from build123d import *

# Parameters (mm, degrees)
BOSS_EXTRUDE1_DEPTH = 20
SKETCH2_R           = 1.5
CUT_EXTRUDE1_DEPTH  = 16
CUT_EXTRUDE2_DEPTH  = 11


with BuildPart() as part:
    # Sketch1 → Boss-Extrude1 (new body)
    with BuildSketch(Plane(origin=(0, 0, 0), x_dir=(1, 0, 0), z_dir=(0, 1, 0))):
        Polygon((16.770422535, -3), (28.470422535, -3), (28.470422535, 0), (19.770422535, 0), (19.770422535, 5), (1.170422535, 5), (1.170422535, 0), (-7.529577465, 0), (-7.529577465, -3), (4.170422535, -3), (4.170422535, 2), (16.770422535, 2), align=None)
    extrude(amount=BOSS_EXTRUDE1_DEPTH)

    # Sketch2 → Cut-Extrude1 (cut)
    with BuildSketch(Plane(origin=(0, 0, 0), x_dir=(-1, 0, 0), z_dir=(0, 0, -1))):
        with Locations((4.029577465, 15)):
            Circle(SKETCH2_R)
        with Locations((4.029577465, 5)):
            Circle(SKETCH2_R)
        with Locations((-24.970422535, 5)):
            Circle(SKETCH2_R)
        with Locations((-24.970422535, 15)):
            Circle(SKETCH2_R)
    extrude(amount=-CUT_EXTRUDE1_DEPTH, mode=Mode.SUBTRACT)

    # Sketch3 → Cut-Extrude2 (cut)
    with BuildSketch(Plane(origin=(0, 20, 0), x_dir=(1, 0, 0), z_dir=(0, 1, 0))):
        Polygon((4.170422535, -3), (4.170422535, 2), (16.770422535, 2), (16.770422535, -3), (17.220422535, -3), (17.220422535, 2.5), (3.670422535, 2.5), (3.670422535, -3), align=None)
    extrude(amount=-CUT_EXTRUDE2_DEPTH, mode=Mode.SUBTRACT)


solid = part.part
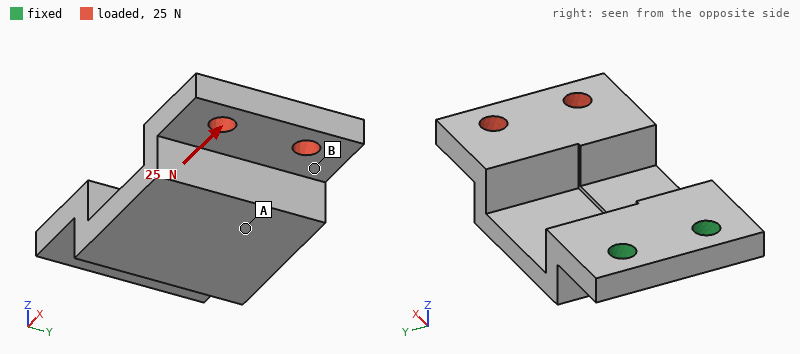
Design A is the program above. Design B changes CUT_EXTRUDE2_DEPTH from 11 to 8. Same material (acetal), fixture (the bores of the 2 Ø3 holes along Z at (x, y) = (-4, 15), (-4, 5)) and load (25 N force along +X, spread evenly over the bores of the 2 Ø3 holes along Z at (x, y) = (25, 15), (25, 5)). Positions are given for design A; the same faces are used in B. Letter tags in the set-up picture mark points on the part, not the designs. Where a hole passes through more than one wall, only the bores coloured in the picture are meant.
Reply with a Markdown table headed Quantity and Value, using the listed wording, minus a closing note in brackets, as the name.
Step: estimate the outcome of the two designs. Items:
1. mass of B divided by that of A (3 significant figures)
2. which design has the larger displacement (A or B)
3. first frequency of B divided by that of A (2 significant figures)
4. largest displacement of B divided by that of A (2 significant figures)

| Quantity | Value |
|---|---|
| mass of B divided by that of A | 1.01 |
| which design has the larger displacement | A |
| first frequency of B divided by that of A | 1.0 |
| largest displacement of B divided by that of A | 0.90 |
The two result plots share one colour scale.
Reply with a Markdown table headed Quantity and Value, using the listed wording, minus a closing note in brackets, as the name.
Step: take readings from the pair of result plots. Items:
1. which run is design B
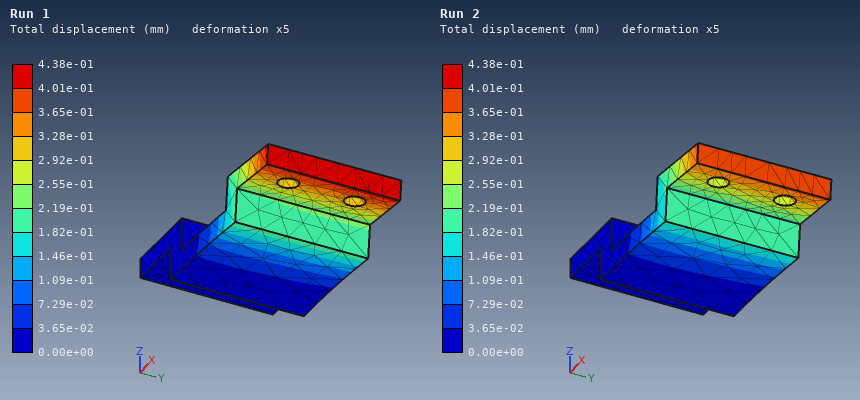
| Quantity | Value |
|---|---|
| which run is design B | Run 2 |
